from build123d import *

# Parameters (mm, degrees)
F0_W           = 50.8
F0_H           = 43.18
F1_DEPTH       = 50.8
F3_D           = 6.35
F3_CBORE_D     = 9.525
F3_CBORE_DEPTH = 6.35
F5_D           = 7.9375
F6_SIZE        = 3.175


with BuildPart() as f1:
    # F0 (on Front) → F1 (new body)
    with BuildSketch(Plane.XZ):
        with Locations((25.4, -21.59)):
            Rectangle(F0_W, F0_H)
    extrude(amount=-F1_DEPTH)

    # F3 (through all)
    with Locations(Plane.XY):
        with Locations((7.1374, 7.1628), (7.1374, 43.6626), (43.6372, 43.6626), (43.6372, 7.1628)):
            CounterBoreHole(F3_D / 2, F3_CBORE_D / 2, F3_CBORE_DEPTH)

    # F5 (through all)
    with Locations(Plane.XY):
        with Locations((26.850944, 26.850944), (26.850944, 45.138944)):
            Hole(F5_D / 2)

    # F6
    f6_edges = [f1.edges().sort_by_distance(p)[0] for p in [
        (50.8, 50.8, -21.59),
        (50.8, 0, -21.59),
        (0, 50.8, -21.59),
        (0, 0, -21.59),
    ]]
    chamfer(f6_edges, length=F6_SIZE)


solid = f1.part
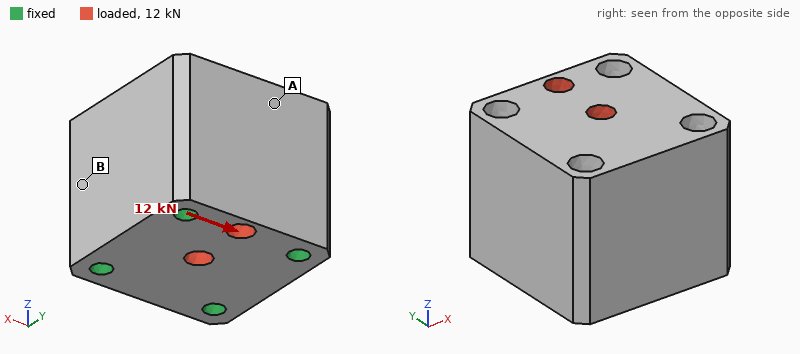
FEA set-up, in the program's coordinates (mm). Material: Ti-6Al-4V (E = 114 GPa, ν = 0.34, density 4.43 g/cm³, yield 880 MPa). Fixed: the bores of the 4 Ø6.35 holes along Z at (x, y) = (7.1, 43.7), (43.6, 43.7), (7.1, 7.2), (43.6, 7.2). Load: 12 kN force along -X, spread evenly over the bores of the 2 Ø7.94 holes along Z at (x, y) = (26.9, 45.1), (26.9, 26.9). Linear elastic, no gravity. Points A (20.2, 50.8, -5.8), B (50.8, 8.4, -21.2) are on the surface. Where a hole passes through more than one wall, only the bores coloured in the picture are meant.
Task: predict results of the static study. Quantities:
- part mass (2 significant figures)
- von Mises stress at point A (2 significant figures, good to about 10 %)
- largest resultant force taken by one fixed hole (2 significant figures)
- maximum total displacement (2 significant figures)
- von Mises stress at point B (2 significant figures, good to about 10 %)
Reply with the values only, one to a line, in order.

440 g
5.9 MPa
4.6 kN
1.3 µm
2.2 MPa
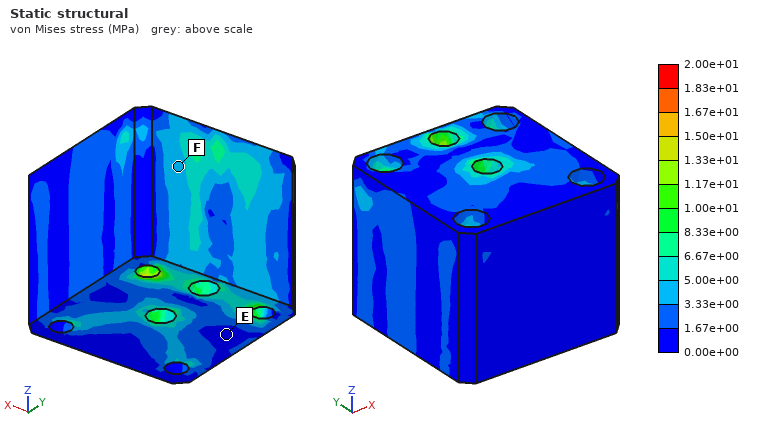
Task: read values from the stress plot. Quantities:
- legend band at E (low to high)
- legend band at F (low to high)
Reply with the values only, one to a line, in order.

0.00e+00 to 1.67e+00 MPa
3.33e+00 to 5.00e+00 MPa
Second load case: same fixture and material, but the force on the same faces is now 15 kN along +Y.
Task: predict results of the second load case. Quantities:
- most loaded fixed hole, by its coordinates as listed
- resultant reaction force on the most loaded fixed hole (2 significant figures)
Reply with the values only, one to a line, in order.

(43.6, 43.7)
4.9 kN
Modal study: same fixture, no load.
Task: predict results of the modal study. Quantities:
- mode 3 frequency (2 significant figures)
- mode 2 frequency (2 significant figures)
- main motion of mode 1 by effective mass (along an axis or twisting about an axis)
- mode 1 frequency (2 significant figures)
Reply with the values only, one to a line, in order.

37 kHz
35 kHz
along Z
32 kHz
